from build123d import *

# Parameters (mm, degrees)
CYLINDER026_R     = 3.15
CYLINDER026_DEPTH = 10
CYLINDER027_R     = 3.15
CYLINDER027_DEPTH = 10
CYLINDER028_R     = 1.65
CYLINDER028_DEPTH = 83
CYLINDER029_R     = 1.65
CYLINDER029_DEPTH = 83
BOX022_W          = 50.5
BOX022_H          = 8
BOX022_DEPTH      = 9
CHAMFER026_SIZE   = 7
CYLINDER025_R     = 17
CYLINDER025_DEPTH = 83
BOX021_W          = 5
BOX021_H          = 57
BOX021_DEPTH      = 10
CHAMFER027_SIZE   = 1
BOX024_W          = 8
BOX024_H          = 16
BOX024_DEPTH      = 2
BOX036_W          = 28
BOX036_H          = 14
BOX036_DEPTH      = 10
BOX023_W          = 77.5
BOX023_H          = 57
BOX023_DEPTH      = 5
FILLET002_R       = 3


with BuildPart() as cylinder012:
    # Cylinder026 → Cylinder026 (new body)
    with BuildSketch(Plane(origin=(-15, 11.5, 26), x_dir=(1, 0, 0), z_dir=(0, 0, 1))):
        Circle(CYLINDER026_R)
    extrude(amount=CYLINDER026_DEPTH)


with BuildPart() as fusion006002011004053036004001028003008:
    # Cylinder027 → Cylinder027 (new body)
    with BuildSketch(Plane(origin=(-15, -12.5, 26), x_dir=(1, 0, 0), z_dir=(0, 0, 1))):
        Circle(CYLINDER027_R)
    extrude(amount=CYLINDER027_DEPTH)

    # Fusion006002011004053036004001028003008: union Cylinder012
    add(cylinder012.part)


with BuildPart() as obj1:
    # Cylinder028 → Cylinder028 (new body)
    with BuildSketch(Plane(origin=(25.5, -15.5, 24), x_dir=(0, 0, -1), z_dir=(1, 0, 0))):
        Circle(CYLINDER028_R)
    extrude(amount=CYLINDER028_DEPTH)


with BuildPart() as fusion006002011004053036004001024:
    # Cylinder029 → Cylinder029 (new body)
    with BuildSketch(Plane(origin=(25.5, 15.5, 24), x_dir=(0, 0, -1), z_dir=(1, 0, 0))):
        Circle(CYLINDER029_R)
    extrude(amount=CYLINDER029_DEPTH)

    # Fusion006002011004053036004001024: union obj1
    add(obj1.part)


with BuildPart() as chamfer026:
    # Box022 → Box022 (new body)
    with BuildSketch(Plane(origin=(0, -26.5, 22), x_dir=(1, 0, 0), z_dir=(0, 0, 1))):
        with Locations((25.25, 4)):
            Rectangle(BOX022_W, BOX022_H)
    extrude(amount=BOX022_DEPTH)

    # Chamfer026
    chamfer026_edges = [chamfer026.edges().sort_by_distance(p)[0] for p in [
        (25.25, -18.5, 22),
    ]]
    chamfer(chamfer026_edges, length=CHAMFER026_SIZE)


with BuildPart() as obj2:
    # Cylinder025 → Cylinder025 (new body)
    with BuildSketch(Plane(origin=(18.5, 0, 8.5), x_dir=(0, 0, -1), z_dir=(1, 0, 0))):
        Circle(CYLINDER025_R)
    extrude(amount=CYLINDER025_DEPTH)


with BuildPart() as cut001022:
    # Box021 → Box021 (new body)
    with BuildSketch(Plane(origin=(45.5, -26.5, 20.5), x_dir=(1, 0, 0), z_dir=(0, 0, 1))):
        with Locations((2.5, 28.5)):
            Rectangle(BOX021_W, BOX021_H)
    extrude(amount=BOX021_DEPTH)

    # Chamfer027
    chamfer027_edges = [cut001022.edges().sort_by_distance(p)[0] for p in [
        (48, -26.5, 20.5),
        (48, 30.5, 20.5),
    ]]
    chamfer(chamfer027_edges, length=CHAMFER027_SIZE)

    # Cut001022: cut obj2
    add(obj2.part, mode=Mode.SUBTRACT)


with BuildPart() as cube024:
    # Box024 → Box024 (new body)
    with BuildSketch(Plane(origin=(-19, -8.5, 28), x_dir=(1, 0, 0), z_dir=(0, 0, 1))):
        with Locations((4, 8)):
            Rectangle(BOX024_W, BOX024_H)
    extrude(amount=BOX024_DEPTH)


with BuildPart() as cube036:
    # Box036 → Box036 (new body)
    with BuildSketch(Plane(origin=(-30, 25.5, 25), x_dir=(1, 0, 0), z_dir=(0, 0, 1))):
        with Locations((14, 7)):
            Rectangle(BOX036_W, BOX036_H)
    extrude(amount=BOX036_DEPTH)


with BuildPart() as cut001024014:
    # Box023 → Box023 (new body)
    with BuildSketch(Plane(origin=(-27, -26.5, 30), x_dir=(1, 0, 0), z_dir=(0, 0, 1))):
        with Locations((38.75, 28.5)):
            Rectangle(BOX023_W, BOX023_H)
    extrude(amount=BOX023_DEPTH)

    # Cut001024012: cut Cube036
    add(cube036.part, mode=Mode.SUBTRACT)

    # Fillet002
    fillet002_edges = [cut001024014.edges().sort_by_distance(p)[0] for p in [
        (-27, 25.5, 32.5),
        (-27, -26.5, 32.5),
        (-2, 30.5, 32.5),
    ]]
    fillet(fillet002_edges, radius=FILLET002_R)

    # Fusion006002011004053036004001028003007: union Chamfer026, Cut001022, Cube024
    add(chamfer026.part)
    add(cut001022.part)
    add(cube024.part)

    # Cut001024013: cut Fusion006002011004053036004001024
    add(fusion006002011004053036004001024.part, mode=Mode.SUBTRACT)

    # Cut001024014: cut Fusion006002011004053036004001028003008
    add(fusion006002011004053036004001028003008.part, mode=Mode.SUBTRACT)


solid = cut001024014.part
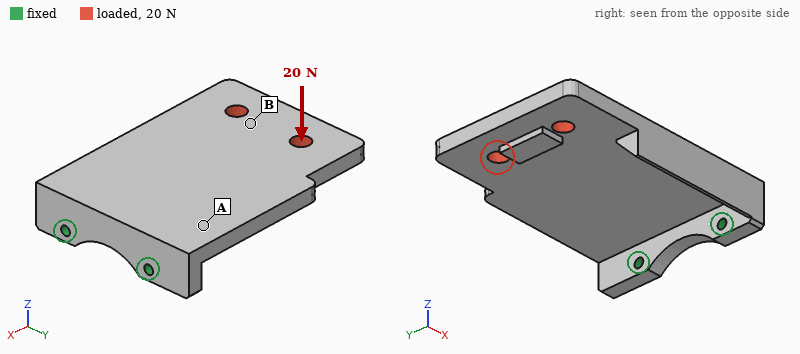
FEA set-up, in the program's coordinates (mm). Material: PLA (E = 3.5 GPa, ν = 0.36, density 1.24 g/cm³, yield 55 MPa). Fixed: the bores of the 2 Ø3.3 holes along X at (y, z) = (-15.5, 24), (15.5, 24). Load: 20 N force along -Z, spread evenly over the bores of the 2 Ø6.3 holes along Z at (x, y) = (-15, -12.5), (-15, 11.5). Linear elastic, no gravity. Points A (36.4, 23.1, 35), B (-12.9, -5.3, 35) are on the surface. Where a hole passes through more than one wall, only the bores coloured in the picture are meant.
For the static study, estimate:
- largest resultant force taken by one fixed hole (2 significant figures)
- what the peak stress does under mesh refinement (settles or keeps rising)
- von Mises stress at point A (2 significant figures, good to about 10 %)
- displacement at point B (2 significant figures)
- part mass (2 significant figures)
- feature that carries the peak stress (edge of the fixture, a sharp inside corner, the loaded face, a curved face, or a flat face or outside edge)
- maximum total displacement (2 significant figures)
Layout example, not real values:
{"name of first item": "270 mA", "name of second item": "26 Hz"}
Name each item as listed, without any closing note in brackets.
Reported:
{"largest resultant force taken by one fixed hole": "12 N", "what the peak stress does under mesh refinement": "keeps rising", "von Mises stress at point A": "2.7 MPa", "displacement at point B": "0.79 mm", "part mass": "31 g", "feature that carries the peak stress": "edge of the fixture", "maximum total displacement": "1.1 mm"}
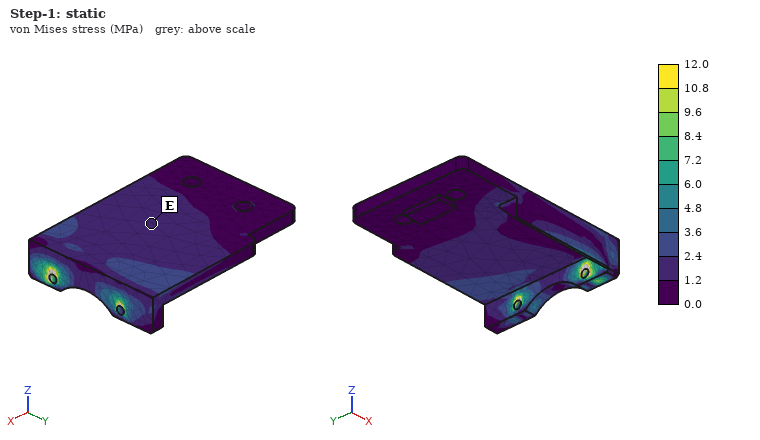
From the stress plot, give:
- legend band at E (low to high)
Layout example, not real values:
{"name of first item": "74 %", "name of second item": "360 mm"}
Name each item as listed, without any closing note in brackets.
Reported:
{"legend band at E": "1.2 to 2.4 MPa"}
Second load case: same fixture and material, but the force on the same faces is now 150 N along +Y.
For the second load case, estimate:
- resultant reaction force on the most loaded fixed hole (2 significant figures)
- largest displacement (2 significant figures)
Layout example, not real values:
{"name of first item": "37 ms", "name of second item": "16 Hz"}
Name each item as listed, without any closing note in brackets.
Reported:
{"resultant reaction force on the most loaded fixed hole": "280 N", "largest displacement": "0.72 mm"}
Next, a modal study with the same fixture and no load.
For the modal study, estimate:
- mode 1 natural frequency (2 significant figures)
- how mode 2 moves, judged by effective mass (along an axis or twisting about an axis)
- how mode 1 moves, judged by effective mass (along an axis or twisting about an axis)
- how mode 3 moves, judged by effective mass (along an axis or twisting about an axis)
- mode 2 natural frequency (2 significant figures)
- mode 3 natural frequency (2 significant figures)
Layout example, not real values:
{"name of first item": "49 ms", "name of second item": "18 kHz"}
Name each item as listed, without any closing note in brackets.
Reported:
{"mode 1 natural frequency": "230 Hz", "how mode 2 moves, judged by effective mass": "along Y", "how mode 1 moves, judged by effective mass": "along Z", "how mode 3 moves, judged by effective mass": "along Y", "mode 2 natural frequency": "690 Hz", "mode 3 natural frequency": "1000 Hz"}
